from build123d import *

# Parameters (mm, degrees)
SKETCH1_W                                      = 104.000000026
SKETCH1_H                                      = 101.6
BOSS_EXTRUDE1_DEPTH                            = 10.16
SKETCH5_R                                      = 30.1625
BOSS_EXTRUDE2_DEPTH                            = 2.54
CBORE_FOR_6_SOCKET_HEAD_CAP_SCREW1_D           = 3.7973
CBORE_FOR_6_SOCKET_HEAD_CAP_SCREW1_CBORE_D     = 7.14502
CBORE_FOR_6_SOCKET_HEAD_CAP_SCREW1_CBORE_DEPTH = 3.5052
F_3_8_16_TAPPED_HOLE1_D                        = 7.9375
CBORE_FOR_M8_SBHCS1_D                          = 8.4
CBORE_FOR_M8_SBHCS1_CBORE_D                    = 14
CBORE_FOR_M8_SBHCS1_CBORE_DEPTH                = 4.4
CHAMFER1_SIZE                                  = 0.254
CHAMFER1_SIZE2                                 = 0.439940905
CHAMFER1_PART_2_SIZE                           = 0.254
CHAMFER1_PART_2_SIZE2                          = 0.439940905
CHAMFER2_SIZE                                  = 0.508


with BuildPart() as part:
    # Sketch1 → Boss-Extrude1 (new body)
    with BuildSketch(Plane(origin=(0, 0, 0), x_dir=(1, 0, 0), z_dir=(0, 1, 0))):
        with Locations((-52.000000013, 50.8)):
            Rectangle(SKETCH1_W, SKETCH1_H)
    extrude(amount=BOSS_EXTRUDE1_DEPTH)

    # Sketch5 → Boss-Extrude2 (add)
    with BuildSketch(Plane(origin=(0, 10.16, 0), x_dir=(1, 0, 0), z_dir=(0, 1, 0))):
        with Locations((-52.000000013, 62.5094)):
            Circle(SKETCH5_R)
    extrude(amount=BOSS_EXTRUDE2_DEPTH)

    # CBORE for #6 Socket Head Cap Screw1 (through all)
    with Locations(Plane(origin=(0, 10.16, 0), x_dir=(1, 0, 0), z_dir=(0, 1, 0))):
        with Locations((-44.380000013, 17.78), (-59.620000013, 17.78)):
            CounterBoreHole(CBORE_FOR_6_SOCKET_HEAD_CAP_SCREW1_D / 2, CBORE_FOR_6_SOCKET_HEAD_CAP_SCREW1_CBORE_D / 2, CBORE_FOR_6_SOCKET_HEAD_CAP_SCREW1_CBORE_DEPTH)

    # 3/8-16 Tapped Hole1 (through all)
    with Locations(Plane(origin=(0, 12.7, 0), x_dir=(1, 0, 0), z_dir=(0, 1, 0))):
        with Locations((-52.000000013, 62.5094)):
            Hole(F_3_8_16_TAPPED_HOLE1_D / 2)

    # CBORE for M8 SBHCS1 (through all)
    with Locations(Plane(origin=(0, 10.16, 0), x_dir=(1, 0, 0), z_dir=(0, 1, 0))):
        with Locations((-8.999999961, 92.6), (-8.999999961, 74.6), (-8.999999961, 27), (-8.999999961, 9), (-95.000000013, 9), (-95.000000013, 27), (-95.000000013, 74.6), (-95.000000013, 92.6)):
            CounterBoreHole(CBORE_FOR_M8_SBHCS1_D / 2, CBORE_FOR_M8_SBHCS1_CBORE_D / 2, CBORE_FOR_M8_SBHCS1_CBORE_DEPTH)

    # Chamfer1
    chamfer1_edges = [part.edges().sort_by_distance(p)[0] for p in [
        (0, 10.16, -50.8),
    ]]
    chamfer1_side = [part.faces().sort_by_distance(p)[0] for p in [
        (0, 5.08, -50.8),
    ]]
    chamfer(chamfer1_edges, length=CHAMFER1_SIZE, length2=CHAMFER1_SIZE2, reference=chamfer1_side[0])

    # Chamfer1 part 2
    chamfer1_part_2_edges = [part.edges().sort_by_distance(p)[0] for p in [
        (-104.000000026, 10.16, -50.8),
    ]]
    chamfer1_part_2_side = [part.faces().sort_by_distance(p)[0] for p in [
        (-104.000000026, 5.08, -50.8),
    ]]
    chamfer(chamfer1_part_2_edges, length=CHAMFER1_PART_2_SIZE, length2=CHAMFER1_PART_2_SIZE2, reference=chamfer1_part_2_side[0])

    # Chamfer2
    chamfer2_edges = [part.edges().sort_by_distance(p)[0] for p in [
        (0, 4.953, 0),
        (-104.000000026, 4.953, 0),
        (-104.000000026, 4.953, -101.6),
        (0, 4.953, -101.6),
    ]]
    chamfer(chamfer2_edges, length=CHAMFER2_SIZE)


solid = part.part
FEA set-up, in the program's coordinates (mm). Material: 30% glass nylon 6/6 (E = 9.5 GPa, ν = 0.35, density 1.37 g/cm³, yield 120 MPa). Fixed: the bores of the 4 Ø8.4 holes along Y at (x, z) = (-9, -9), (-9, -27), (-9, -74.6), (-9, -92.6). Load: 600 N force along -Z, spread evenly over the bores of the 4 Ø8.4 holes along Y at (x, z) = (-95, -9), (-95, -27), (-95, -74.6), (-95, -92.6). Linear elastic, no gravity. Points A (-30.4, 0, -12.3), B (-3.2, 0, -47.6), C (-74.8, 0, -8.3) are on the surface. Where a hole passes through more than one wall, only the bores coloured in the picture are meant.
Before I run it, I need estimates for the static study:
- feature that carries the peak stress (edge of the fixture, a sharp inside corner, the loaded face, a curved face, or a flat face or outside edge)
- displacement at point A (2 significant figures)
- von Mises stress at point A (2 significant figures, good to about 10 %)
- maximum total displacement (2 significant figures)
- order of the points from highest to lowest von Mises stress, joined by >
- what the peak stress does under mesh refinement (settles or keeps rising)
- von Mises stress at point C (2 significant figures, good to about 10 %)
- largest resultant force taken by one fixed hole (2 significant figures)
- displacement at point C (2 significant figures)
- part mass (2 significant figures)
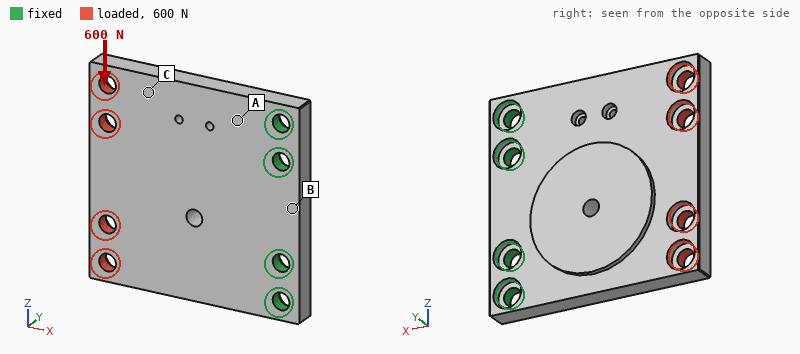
edge of the fixture
14 µm
2.5 MPa
83 µm
A > C > B
keeps rising
1.4 MPa
490 N
51 µm
140 g
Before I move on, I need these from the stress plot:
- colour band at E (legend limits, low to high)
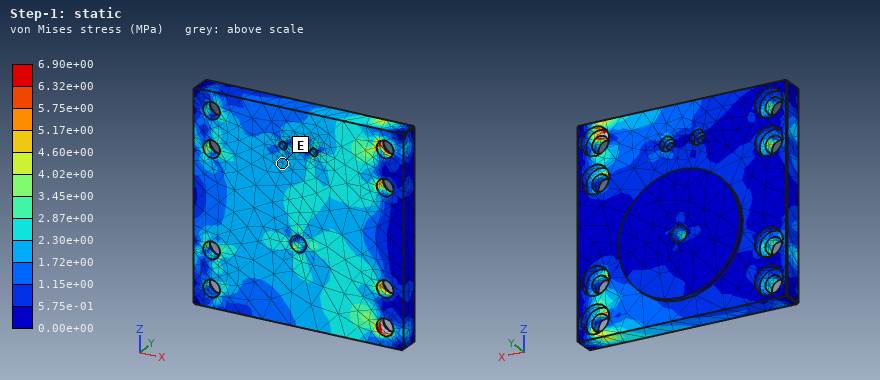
1.72e+00 to 2.30e+00 MPa
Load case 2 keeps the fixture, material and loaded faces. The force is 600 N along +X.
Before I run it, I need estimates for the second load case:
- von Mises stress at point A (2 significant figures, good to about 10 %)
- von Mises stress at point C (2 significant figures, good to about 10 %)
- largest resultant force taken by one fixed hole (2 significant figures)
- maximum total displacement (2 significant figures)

1.4 MPa
1.6 MPa
170 N
58 µm
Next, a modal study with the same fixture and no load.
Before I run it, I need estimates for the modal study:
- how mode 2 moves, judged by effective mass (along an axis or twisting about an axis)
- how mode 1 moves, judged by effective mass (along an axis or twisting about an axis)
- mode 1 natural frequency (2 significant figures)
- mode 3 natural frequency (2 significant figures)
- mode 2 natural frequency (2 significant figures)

twisting about X
along Y
430 Hz
2800 Hz
1200 Hz
